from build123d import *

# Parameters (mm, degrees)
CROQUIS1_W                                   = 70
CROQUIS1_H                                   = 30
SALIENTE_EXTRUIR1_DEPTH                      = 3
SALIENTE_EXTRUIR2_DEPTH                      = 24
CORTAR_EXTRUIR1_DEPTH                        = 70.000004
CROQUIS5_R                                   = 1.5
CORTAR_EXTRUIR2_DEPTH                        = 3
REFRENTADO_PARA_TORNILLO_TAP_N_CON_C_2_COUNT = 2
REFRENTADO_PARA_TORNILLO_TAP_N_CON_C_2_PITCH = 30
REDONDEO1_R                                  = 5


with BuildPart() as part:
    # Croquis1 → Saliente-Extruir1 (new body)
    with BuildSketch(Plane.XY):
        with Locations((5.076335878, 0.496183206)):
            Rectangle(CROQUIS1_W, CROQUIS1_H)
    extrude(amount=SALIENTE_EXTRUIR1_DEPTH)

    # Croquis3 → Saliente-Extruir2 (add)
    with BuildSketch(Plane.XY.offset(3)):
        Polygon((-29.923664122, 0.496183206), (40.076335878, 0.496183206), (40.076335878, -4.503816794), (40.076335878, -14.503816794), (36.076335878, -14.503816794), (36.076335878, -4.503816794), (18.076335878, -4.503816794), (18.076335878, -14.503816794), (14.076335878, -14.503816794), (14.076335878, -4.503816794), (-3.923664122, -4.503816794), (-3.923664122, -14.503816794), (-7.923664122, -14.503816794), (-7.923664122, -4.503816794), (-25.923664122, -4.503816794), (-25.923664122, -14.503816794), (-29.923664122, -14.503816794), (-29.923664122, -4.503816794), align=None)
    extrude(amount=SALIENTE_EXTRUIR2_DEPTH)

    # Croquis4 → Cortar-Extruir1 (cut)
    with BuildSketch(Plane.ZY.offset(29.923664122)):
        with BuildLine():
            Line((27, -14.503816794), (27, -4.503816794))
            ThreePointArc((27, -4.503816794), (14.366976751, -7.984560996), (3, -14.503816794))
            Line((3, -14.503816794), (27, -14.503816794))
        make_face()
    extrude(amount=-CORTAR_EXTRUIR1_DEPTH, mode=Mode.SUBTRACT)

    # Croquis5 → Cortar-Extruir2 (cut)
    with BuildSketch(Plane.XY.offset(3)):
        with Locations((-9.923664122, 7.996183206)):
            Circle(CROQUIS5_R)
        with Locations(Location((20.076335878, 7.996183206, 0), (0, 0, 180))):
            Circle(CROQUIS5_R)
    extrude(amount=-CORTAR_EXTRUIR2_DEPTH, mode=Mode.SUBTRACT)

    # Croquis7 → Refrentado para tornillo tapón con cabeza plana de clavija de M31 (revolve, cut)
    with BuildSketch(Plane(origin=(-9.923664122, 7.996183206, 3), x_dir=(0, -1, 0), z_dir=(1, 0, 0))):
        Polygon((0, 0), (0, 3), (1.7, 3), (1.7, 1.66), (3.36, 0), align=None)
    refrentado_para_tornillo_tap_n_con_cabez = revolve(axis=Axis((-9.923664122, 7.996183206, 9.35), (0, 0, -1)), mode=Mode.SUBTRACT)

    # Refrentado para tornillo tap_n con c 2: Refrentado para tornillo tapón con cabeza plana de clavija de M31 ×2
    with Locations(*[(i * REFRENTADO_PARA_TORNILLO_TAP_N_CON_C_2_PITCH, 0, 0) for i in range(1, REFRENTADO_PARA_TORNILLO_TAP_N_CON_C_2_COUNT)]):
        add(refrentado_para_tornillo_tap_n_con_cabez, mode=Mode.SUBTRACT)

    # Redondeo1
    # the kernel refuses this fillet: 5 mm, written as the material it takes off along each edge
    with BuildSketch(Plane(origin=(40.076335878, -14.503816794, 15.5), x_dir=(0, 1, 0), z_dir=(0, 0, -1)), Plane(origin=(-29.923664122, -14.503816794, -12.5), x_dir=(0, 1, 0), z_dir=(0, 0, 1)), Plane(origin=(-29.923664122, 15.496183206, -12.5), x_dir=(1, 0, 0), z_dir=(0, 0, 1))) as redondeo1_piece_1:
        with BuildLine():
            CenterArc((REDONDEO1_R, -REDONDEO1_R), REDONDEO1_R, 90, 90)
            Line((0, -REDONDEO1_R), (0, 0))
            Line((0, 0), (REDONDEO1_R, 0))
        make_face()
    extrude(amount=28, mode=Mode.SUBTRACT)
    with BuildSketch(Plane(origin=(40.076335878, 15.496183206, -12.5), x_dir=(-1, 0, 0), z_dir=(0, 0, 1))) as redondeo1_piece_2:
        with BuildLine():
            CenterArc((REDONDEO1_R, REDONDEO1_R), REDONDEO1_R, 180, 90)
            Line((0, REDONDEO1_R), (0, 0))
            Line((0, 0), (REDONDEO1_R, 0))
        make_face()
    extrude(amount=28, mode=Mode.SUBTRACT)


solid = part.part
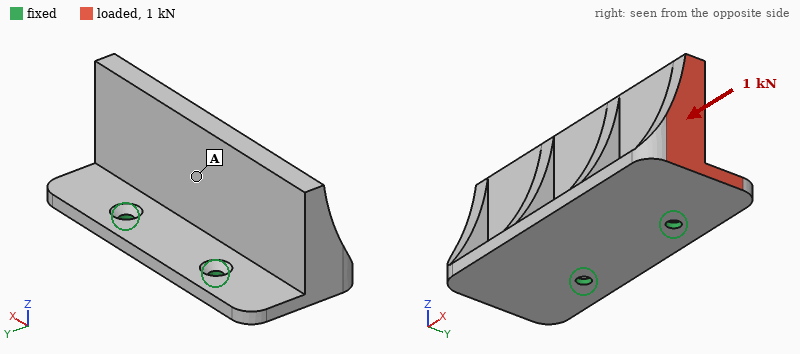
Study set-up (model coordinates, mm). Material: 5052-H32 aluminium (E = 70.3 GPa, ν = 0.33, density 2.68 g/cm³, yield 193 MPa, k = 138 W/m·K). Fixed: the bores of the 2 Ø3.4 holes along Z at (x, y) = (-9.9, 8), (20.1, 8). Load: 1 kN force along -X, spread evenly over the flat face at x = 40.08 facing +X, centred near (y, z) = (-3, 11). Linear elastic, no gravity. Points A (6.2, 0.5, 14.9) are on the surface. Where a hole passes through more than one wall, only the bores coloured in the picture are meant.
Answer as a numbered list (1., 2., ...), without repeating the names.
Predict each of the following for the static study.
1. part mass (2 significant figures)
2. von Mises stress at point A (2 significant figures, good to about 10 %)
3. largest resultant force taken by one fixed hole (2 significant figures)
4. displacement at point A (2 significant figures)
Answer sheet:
1. 43 g
2. 9.8 MPa
3. 710 N
4. 19 µm
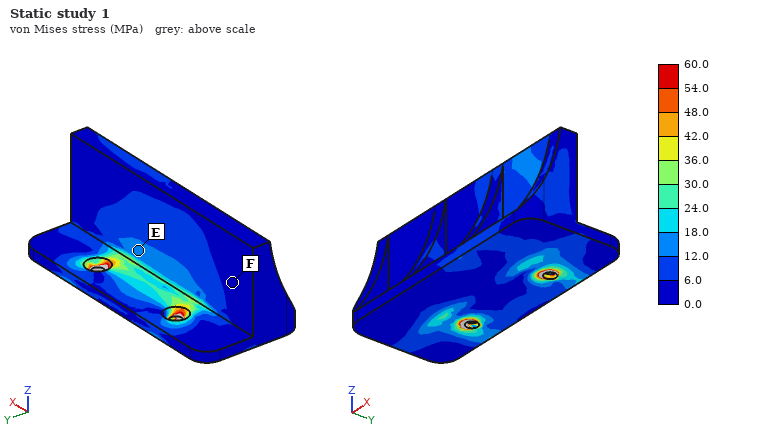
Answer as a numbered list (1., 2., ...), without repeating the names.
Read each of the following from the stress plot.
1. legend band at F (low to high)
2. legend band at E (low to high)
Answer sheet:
1. 0.0 to 6.0 MPa
2. 12.0 to 18.0 MPa
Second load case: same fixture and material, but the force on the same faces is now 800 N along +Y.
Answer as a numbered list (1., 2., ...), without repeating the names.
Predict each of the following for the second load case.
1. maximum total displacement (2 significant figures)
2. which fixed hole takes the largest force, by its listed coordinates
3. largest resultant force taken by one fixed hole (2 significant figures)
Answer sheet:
1. 0.50 mm
2. (20.1, 8)
3. 1.3 kN
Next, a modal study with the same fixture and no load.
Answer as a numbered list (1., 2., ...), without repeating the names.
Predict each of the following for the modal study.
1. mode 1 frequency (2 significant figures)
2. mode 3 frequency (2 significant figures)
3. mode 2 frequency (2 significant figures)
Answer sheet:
1. 1200 Hz
2. 5700 Hz
3. 2900 Hz
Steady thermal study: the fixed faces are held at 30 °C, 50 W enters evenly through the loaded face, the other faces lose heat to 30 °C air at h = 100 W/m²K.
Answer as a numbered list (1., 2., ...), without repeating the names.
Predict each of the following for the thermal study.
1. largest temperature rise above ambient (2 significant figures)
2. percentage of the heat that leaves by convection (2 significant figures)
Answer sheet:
1. 63 K
2. 37 %
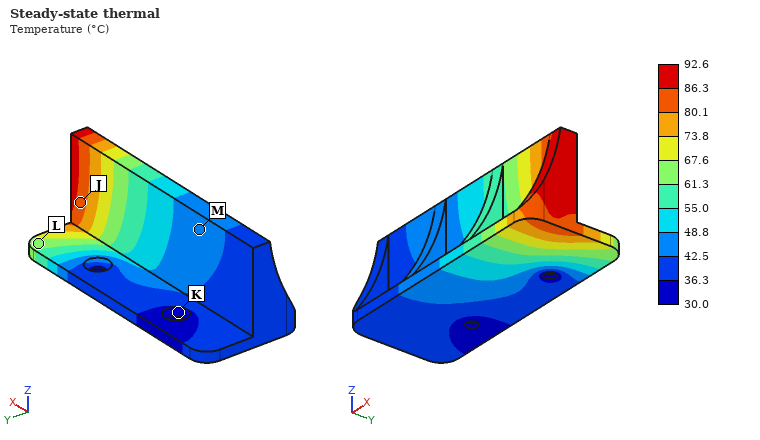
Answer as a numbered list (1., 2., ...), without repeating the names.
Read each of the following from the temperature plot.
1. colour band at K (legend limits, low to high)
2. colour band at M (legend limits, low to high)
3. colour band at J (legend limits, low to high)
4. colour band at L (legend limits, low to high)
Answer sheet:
1. 30.0 to 36.3 °C
2. 42.5 to 48.8 °C
3. 80.1 to 86.3 °C
4. 61.3 to 67.6 °C
